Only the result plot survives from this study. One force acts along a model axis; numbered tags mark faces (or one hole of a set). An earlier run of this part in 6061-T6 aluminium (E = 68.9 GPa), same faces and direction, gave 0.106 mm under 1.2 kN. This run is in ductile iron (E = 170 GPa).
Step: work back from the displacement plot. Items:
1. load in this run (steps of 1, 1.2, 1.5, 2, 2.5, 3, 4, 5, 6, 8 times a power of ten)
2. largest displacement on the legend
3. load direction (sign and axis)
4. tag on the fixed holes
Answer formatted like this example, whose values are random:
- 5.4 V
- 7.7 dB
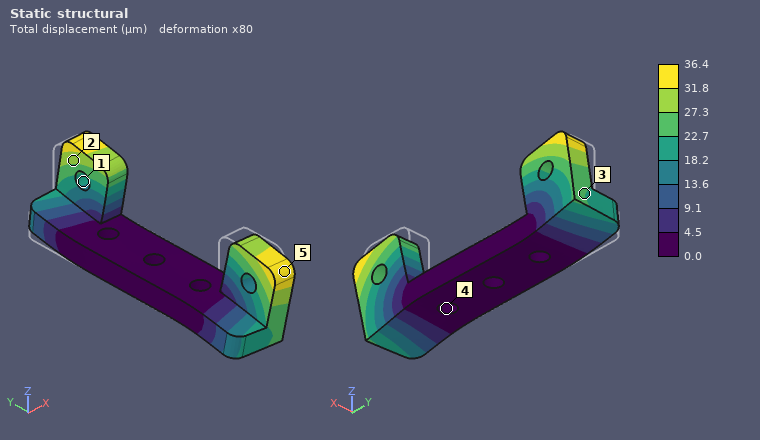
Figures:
- 1 kN
- 36.4 µm
- -Y
- 4
